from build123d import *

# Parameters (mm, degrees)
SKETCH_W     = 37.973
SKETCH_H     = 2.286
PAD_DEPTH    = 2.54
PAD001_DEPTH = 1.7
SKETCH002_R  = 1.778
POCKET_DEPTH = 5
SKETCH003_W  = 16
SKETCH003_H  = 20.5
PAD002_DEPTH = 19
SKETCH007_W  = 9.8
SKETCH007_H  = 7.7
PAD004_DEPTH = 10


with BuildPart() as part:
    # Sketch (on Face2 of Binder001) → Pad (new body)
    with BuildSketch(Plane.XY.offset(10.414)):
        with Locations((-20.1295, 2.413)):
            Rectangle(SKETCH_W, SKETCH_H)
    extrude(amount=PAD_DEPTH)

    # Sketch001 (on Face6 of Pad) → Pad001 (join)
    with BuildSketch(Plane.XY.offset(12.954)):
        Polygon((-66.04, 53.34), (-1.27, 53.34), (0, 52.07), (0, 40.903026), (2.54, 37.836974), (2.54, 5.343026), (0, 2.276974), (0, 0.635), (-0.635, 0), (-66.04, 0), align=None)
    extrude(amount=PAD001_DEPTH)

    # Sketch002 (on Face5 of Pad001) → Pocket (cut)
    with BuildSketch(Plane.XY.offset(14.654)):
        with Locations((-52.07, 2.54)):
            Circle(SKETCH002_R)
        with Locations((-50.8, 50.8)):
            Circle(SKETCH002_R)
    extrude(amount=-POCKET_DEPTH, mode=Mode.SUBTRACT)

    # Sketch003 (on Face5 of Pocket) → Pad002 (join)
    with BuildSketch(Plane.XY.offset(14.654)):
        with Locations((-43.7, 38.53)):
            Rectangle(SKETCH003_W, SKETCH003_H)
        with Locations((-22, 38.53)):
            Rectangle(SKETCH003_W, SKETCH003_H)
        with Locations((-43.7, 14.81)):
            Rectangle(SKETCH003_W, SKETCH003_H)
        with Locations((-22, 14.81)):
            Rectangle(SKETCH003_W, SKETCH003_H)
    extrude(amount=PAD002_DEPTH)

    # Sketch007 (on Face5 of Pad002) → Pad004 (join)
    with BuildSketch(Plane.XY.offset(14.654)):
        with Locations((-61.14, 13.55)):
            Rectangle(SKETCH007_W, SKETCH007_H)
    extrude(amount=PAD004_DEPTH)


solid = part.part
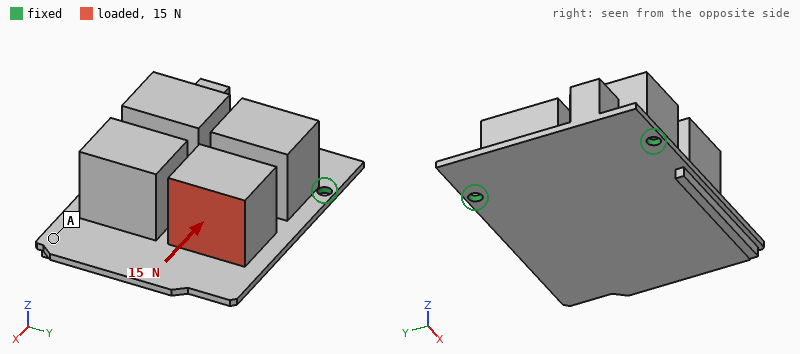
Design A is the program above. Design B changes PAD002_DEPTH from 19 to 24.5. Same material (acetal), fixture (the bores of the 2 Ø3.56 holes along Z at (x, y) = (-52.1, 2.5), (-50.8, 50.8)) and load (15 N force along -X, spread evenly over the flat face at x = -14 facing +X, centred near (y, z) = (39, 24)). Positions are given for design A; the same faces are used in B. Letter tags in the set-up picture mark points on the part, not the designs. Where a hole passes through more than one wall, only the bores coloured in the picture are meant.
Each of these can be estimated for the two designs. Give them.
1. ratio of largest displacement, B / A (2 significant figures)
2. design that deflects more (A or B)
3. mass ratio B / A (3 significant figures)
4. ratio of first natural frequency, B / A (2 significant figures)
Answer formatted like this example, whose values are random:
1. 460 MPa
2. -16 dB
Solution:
1. 1.2
2. B
3. 1.23
4. 0.86
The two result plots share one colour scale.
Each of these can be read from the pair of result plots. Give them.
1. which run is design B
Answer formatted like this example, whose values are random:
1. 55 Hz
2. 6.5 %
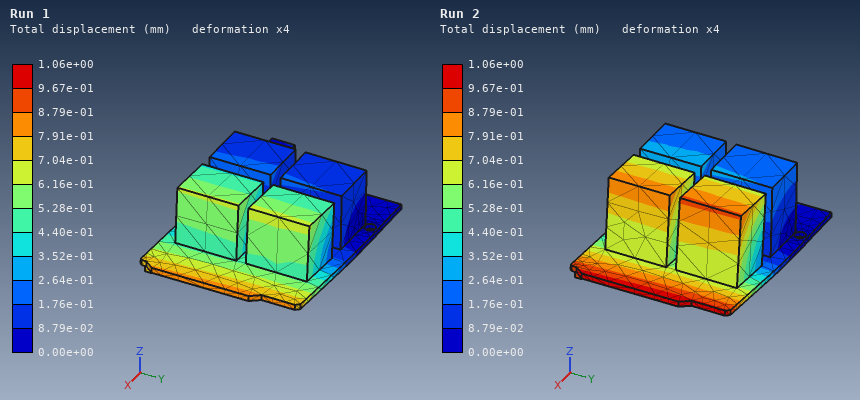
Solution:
1. Run 2
